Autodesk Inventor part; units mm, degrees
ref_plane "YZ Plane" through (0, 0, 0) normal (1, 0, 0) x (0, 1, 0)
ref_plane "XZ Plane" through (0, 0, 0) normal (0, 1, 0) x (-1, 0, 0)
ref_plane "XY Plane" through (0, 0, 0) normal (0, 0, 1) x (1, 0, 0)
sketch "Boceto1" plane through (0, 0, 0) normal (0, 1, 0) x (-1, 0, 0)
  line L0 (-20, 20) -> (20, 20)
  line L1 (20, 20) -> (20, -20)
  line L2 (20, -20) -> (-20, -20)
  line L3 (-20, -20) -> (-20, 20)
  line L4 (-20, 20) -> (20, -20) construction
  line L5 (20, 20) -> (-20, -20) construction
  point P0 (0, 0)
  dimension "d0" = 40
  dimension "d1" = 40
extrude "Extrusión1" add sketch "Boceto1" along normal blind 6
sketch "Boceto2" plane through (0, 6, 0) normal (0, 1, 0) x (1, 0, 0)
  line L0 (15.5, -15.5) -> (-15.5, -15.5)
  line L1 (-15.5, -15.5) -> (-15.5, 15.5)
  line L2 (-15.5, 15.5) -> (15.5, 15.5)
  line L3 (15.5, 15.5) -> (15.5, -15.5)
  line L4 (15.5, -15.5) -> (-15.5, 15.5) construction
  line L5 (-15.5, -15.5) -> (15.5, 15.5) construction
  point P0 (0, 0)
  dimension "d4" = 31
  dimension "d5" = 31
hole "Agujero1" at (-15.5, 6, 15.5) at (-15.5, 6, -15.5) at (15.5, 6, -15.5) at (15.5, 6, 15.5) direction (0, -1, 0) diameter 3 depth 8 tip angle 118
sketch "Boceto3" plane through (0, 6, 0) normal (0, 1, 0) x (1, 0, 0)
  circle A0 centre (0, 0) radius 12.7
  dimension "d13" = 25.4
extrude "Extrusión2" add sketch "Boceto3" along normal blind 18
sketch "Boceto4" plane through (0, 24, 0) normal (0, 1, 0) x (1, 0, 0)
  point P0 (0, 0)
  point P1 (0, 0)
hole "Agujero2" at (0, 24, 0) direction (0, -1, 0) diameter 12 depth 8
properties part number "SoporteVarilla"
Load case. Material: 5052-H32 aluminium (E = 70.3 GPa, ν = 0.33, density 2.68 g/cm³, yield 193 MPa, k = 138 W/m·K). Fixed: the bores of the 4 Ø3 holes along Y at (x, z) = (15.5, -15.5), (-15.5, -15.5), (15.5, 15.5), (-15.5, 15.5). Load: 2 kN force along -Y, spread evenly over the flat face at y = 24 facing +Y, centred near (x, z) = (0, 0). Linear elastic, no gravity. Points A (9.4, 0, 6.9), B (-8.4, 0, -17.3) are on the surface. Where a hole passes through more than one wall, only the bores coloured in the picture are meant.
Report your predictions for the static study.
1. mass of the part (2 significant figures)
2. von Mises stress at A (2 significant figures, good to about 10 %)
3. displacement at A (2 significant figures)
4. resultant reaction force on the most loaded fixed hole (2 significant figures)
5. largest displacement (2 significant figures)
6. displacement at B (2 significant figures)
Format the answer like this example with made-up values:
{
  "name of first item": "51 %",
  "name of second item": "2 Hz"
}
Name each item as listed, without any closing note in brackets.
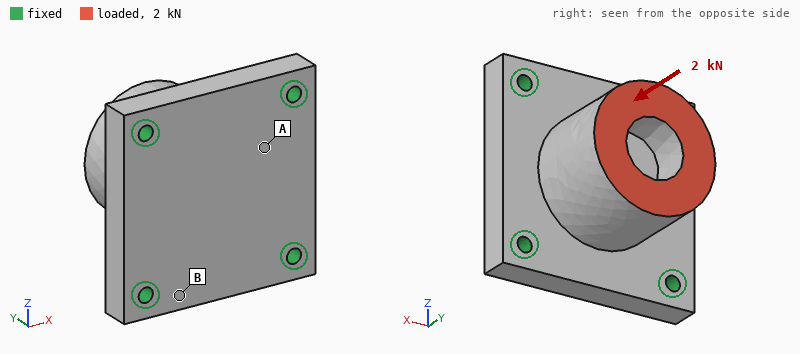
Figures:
{
  "mass of the part": "47 g",
  "von Mises stress at A": "12 MPa",
  "displacement at A": "6.1 µm",
  "resultant reaction force on the most loaded fixed hole": "510 N",
  "largest displacement": "8.0 µm",
  "displacement at B": "3.1 µm"
}
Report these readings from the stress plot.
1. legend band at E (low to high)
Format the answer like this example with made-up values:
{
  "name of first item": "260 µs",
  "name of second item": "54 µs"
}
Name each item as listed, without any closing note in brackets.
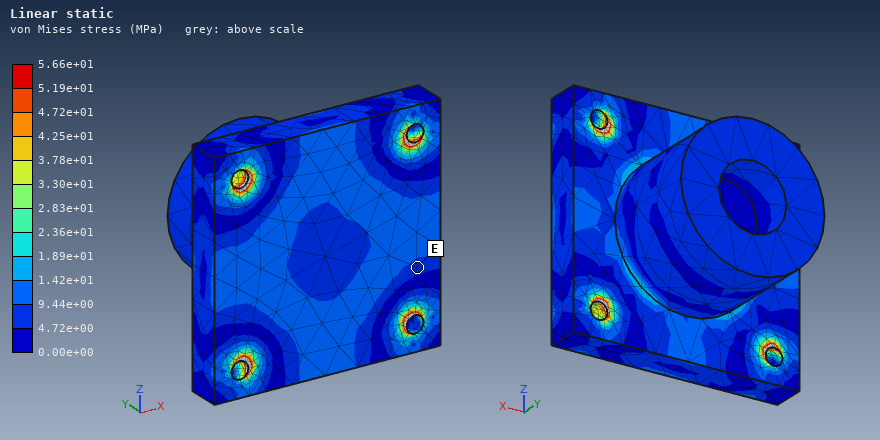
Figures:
{
  "legend band at E": "4.72e+00 to 9.44e+00 MPa"
}
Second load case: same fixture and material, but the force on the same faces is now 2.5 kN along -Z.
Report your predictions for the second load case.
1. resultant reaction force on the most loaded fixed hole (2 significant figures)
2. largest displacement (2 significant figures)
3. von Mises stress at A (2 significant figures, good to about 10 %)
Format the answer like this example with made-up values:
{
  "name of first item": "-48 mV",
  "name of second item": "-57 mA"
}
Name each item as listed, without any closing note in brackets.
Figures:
{
  "resultant reaction force on the most loaded fixed hole": "1.2 kN",
  "largest displacement": "37 µm",
  "von Mises stress at A": "24 MPa"
}
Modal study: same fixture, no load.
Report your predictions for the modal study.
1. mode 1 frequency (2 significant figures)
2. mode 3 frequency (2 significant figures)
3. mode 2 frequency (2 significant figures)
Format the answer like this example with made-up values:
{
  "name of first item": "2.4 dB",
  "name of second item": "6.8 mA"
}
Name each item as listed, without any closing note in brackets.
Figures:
{
  "mode 1 frequency": "14 kHz",
  "mode 3 frequency": "14 kHz",
  "mode 2 frequency": "14 kHz"
}
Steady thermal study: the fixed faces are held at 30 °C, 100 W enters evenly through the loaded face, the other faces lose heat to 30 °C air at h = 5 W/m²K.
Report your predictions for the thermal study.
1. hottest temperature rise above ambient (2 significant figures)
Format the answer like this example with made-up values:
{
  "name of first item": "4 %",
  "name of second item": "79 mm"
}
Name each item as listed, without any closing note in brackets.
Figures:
{
  "hottest temperature rise above ambient": "55 K"
}
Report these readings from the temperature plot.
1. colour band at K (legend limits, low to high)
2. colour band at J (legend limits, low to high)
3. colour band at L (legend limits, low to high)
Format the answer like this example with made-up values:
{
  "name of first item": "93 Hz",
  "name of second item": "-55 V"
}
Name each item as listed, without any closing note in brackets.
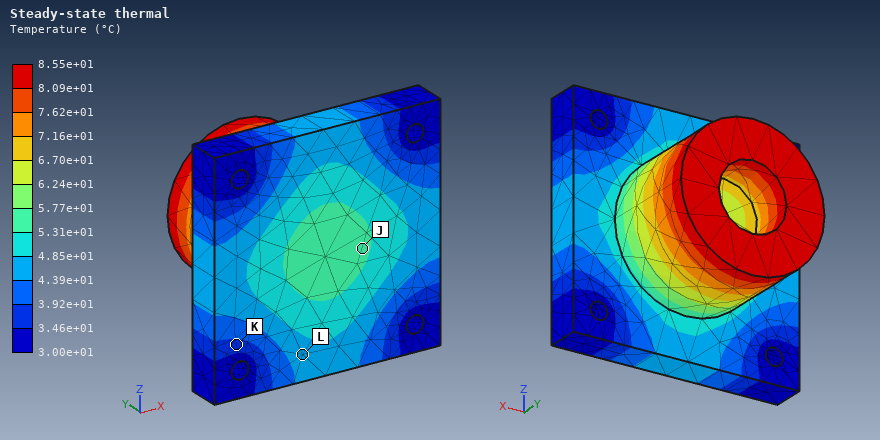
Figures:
{
  "colour band at K": "3.46e+01 to 3.92e+01 °C",
  "colour band at J": "5.31e+01 to 5.77e+01 °C",
  "colour band at L": "4.39e+01 to 4.85e+01 °C"
}
